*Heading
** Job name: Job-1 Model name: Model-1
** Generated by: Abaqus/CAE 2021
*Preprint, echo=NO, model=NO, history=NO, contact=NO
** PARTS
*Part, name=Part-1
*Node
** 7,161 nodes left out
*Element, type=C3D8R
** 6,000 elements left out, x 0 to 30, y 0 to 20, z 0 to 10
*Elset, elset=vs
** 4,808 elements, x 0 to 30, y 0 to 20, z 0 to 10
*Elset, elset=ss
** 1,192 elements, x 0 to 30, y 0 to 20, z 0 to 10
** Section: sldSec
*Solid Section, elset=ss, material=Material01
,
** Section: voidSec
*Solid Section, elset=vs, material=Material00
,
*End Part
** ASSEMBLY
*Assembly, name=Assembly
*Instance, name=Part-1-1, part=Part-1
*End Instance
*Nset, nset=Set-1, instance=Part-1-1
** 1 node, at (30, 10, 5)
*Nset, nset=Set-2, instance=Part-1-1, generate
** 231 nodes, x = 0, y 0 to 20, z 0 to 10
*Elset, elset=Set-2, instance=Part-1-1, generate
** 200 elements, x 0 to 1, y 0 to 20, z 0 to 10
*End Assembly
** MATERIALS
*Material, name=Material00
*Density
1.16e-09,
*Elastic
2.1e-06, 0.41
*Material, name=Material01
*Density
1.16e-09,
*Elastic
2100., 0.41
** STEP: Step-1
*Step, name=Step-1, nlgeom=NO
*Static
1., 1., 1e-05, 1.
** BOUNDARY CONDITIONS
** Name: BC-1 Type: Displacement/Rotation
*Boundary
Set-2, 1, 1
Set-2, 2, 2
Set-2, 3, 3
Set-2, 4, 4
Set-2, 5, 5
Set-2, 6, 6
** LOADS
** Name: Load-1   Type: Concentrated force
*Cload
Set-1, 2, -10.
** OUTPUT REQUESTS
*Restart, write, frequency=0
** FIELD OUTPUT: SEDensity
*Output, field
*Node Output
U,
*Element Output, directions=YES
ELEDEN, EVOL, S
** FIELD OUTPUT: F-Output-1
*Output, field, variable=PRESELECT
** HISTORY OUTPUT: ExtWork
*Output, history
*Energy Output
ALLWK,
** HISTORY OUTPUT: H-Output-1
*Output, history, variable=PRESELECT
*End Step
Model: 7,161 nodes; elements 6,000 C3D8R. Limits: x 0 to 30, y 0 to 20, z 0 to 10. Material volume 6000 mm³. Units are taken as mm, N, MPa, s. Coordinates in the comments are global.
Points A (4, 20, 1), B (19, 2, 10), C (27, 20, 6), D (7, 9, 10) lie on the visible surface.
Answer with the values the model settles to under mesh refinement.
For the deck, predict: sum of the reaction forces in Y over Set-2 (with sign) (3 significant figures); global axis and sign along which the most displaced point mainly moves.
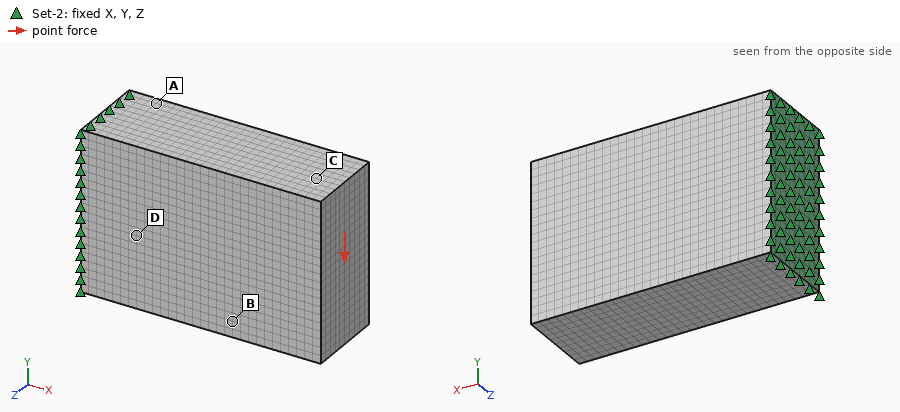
10.0 N
-Y
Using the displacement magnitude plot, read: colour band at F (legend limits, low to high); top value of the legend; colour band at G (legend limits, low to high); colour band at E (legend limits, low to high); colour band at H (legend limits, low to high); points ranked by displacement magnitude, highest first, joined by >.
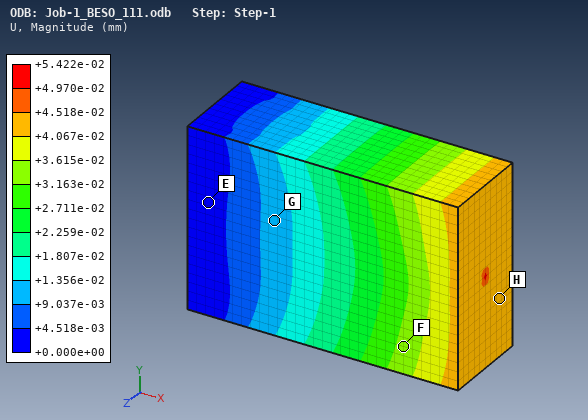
+3.163e-02 to +3.615e-02 mm
+5.422e-02 mm
+9.037e-03 to +1.356e-02 mm
+0.000e+00 to +4.518e-03 mm
+4.067e-02 to +4.518e-02 mm
H > F > G > E
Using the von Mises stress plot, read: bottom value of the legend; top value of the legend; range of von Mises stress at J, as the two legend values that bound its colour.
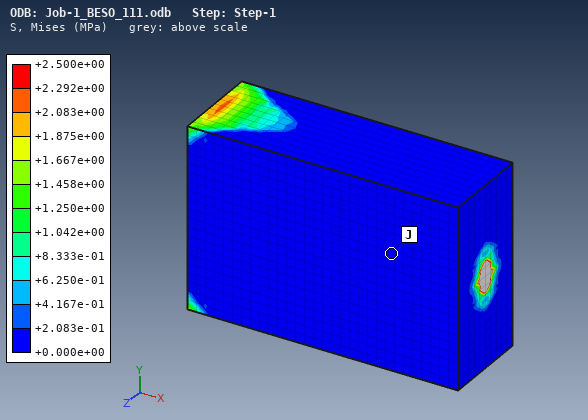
+0.000e+00 MPa
+2.500e+00 MPa
+0.000e+00 to +2.083e-01 MPa
